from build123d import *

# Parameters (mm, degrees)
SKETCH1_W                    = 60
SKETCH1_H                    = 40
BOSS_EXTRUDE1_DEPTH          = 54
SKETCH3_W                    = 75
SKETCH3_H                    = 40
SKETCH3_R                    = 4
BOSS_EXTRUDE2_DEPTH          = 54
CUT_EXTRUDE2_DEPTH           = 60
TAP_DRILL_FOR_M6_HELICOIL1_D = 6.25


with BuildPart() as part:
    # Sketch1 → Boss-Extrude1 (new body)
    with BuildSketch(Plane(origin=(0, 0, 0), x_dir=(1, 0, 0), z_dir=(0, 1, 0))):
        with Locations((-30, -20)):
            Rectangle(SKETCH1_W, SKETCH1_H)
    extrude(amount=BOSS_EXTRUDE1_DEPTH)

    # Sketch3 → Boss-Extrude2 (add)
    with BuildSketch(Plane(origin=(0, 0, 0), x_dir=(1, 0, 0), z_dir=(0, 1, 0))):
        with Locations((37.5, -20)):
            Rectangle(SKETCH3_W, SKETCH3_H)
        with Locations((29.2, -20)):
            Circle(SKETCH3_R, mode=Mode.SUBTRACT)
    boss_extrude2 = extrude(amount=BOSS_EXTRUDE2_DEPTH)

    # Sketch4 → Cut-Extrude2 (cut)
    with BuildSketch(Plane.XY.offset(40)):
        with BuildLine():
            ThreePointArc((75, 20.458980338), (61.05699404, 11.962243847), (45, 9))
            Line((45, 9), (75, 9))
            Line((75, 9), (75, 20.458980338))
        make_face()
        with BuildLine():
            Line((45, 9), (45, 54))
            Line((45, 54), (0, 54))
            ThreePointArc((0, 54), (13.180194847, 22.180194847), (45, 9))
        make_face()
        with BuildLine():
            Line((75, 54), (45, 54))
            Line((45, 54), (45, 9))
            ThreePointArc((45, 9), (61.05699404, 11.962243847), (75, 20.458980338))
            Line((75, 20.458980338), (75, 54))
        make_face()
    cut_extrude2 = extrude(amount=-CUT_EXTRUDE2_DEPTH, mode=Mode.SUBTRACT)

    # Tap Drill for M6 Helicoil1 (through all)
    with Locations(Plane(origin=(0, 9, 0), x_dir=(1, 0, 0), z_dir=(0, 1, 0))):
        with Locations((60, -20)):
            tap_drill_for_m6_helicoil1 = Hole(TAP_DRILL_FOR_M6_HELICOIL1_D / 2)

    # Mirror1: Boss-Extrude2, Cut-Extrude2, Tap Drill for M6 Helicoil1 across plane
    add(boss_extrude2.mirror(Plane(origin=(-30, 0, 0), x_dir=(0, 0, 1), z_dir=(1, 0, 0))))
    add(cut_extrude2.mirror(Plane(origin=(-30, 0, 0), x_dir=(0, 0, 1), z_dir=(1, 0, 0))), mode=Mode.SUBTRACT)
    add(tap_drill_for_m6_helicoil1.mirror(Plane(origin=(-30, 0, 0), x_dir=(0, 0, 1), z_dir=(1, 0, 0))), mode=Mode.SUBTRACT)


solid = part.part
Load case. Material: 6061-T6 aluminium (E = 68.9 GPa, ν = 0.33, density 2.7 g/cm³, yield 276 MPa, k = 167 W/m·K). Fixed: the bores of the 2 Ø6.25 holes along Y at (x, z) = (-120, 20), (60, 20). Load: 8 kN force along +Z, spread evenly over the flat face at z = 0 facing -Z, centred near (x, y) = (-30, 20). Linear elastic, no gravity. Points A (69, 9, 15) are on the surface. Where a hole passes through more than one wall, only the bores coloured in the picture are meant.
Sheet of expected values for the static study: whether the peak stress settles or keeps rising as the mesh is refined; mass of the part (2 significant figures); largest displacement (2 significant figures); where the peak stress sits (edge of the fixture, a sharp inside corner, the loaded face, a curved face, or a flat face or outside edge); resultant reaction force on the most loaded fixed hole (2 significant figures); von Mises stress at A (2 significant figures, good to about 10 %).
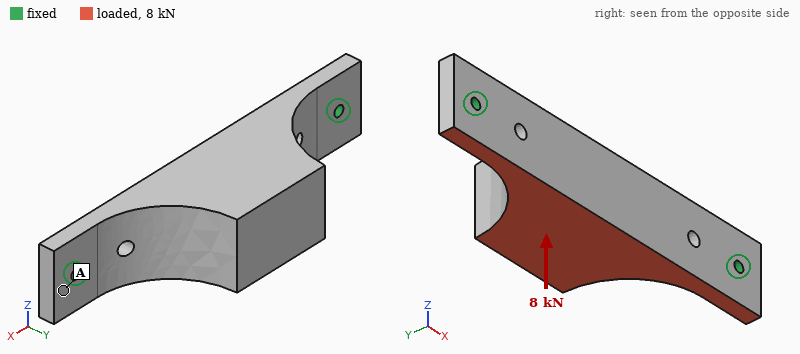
keeps rising
580 g
0.57 mm
edge of the fixture
4.0 kN
38 MPa
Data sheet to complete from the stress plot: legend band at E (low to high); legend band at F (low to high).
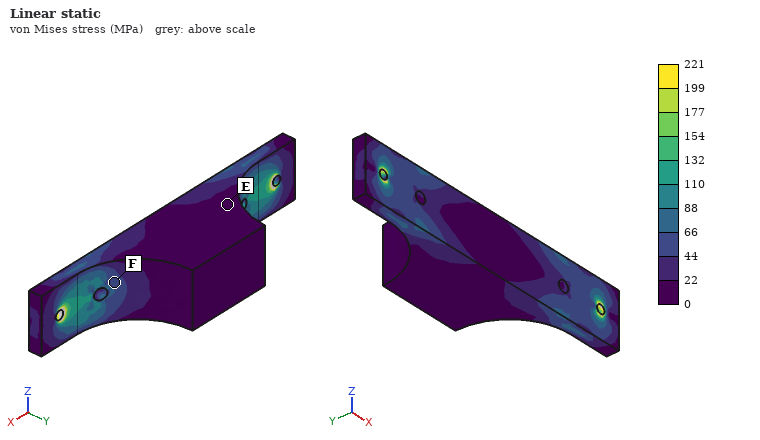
0 to 22 MPa
44 to 66 MPa
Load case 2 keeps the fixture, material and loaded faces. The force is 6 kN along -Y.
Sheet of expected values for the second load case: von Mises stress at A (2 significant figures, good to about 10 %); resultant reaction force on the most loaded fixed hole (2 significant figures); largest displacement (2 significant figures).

36 MPa
4.2 kN
0.46 mm
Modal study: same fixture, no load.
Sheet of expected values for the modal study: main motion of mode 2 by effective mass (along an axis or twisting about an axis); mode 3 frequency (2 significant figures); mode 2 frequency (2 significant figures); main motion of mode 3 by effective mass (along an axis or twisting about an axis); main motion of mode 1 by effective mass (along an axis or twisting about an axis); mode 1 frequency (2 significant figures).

along Y
3200 Hz
1600 Hz
along Z
along Z
930 Hz
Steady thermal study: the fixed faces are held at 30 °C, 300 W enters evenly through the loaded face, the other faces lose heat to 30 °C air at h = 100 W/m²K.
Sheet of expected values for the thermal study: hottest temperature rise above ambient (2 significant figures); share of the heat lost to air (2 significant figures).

75 K
41 %
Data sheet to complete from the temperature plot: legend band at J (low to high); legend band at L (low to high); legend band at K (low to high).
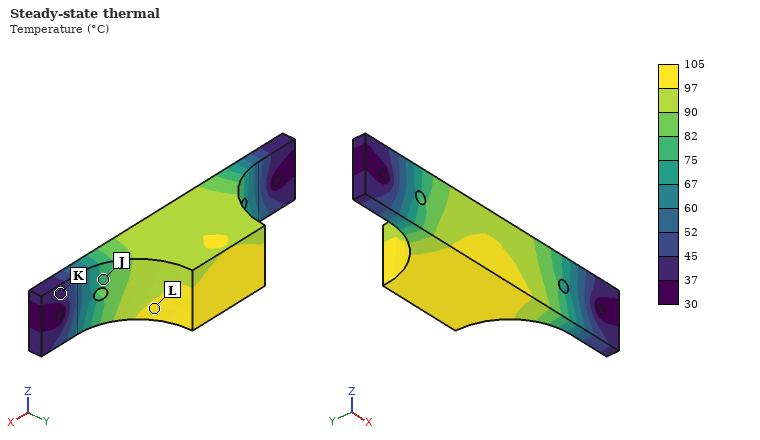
75 to 82 °C
97 to 105 °C
37 to 45 °C
